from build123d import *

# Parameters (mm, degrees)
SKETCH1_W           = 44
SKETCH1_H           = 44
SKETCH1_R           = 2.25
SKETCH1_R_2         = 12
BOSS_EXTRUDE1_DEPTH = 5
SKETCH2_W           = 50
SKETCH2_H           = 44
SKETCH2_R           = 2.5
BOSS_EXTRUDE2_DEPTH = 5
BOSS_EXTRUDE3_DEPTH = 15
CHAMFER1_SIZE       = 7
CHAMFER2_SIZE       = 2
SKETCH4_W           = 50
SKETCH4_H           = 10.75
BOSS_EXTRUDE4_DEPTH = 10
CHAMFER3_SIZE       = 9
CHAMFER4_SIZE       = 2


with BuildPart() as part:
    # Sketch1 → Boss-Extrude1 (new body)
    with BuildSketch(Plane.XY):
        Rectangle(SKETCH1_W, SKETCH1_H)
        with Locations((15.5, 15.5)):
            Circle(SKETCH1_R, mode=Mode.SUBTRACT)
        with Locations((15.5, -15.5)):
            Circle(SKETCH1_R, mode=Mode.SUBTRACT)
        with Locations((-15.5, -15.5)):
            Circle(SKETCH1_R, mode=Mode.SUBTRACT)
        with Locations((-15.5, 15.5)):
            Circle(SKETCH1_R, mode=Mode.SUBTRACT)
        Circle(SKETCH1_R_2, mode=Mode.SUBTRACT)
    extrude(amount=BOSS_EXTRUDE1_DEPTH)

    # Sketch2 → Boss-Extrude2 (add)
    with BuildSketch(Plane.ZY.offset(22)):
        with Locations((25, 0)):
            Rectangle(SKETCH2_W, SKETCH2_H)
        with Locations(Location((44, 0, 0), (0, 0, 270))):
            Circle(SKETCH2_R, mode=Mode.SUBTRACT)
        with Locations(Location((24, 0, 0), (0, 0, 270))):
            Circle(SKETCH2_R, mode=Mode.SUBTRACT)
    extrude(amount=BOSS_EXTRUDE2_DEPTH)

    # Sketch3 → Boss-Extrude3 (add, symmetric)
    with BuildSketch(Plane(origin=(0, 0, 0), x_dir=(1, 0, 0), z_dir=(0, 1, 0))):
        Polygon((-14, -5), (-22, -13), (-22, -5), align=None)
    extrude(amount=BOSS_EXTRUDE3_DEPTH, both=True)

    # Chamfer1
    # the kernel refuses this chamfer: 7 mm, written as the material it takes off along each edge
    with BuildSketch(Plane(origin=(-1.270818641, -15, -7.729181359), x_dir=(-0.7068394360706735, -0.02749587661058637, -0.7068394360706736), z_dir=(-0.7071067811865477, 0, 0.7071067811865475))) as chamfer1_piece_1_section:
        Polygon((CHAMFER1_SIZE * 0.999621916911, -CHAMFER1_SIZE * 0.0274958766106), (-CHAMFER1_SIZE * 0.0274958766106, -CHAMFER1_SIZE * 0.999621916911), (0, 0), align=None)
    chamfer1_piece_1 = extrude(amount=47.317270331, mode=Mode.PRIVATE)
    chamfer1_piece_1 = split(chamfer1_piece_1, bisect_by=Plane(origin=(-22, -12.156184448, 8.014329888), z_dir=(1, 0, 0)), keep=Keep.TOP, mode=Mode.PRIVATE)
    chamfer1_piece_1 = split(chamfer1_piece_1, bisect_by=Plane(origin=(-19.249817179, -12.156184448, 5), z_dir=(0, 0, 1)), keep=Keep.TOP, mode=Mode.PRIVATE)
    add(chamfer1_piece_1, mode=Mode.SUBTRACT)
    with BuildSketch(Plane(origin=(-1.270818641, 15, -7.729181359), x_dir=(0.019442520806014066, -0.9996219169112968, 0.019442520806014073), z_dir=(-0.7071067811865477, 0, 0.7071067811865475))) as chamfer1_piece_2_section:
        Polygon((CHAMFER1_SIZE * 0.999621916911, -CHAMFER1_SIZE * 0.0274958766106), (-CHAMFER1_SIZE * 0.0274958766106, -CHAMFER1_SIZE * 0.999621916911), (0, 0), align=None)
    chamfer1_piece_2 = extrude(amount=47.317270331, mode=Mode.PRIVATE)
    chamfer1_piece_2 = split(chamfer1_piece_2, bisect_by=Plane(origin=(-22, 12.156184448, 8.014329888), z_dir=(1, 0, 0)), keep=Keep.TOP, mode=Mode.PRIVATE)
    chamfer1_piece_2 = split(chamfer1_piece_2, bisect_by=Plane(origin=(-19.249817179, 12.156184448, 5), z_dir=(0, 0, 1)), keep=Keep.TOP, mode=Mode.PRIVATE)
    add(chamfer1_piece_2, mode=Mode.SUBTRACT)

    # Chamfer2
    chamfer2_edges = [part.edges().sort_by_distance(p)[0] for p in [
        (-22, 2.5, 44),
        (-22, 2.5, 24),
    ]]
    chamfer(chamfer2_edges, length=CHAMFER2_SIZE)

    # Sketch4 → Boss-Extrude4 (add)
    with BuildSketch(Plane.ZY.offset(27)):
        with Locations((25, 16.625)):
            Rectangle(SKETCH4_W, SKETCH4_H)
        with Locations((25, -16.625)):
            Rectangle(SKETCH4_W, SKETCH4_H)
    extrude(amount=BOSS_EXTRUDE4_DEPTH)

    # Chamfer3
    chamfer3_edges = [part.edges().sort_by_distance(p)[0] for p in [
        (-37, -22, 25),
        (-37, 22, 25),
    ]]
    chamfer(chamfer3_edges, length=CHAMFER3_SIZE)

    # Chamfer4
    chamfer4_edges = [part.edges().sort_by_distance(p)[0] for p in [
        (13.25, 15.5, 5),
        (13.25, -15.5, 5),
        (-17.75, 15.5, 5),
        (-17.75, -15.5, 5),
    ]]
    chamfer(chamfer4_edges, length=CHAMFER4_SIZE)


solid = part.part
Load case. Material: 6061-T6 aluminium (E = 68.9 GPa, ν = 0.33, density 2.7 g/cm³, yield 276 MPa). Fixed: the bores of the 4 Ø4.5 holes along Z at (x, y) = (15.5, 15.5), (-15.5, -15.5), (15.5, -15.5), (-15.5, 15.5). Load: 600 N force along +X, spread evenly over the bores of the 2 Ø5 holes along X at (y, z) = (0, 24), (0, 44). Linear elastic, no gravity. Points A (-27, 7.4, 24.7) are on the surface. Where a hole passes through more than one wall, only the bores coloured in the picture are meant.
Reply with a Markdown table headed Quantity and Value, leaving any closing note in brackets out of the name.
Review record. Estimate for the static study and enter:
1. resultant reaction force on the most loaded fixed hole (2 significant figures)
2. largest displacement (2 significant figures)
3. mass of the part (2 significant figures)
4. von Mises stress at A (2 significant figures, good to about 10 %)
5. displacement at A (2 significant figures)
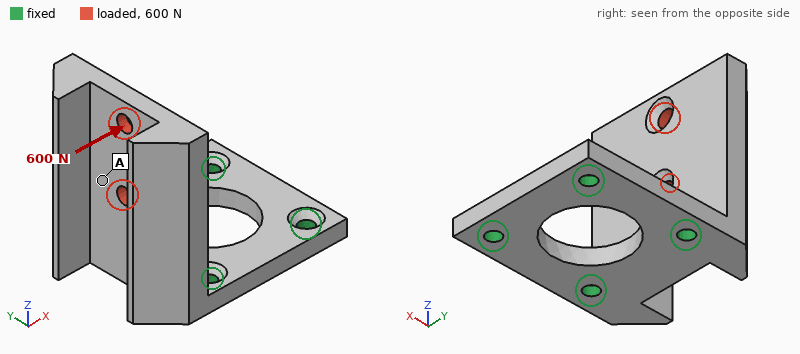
| Quantity | Value |
|---|---|
| resultant reaction force on the most loaded fixed hole | 320 N |
| largest displacement | 0.32 mm |
| mass of the part | 68 g |
| von Mises stress at A | 13 MPa |
| displacement at A | 0.14 mm |
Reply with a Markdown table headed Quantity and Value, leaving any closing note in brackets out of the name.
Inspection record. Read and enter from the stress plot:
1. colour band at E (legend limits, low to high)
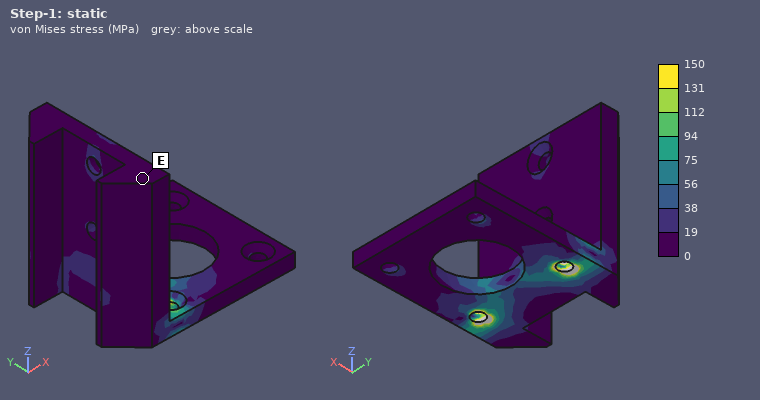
| Quantity | Value |
|---|---|
| colour band at E | 0 to 19 MPa |
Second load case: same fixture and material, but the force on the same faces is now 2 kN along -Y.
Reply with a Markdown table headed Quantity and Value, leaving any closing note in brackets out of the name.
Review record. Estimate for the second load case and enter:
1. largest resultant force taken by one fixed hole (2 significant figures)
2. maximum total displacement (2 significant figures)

| Quantity | Value |
|---|---|
| largest resultant force taken by one fixed hole | 2.4 kN |
| maximum total displacement | 0.10 mm |
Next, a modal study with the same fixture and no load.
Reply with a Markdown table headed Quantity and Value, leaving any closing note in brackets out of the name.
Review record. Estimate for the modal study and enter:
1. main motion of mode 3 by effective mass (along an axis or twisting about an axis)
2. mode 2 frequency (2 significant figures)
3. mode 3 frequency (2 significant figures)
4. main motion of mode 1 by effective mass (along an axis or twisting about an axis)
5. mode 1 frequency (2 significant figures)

| Quantity | Value |
|---|---|
| main motion of mode 3 by effective mass | along Y |
| mode 2 frequency | 4000 Hz |
| mode 3 frequency | 5000 Hz |
| main motion of mode 1 by effective mass | along X |
| mode 1 frequency | 1400 Hz |
